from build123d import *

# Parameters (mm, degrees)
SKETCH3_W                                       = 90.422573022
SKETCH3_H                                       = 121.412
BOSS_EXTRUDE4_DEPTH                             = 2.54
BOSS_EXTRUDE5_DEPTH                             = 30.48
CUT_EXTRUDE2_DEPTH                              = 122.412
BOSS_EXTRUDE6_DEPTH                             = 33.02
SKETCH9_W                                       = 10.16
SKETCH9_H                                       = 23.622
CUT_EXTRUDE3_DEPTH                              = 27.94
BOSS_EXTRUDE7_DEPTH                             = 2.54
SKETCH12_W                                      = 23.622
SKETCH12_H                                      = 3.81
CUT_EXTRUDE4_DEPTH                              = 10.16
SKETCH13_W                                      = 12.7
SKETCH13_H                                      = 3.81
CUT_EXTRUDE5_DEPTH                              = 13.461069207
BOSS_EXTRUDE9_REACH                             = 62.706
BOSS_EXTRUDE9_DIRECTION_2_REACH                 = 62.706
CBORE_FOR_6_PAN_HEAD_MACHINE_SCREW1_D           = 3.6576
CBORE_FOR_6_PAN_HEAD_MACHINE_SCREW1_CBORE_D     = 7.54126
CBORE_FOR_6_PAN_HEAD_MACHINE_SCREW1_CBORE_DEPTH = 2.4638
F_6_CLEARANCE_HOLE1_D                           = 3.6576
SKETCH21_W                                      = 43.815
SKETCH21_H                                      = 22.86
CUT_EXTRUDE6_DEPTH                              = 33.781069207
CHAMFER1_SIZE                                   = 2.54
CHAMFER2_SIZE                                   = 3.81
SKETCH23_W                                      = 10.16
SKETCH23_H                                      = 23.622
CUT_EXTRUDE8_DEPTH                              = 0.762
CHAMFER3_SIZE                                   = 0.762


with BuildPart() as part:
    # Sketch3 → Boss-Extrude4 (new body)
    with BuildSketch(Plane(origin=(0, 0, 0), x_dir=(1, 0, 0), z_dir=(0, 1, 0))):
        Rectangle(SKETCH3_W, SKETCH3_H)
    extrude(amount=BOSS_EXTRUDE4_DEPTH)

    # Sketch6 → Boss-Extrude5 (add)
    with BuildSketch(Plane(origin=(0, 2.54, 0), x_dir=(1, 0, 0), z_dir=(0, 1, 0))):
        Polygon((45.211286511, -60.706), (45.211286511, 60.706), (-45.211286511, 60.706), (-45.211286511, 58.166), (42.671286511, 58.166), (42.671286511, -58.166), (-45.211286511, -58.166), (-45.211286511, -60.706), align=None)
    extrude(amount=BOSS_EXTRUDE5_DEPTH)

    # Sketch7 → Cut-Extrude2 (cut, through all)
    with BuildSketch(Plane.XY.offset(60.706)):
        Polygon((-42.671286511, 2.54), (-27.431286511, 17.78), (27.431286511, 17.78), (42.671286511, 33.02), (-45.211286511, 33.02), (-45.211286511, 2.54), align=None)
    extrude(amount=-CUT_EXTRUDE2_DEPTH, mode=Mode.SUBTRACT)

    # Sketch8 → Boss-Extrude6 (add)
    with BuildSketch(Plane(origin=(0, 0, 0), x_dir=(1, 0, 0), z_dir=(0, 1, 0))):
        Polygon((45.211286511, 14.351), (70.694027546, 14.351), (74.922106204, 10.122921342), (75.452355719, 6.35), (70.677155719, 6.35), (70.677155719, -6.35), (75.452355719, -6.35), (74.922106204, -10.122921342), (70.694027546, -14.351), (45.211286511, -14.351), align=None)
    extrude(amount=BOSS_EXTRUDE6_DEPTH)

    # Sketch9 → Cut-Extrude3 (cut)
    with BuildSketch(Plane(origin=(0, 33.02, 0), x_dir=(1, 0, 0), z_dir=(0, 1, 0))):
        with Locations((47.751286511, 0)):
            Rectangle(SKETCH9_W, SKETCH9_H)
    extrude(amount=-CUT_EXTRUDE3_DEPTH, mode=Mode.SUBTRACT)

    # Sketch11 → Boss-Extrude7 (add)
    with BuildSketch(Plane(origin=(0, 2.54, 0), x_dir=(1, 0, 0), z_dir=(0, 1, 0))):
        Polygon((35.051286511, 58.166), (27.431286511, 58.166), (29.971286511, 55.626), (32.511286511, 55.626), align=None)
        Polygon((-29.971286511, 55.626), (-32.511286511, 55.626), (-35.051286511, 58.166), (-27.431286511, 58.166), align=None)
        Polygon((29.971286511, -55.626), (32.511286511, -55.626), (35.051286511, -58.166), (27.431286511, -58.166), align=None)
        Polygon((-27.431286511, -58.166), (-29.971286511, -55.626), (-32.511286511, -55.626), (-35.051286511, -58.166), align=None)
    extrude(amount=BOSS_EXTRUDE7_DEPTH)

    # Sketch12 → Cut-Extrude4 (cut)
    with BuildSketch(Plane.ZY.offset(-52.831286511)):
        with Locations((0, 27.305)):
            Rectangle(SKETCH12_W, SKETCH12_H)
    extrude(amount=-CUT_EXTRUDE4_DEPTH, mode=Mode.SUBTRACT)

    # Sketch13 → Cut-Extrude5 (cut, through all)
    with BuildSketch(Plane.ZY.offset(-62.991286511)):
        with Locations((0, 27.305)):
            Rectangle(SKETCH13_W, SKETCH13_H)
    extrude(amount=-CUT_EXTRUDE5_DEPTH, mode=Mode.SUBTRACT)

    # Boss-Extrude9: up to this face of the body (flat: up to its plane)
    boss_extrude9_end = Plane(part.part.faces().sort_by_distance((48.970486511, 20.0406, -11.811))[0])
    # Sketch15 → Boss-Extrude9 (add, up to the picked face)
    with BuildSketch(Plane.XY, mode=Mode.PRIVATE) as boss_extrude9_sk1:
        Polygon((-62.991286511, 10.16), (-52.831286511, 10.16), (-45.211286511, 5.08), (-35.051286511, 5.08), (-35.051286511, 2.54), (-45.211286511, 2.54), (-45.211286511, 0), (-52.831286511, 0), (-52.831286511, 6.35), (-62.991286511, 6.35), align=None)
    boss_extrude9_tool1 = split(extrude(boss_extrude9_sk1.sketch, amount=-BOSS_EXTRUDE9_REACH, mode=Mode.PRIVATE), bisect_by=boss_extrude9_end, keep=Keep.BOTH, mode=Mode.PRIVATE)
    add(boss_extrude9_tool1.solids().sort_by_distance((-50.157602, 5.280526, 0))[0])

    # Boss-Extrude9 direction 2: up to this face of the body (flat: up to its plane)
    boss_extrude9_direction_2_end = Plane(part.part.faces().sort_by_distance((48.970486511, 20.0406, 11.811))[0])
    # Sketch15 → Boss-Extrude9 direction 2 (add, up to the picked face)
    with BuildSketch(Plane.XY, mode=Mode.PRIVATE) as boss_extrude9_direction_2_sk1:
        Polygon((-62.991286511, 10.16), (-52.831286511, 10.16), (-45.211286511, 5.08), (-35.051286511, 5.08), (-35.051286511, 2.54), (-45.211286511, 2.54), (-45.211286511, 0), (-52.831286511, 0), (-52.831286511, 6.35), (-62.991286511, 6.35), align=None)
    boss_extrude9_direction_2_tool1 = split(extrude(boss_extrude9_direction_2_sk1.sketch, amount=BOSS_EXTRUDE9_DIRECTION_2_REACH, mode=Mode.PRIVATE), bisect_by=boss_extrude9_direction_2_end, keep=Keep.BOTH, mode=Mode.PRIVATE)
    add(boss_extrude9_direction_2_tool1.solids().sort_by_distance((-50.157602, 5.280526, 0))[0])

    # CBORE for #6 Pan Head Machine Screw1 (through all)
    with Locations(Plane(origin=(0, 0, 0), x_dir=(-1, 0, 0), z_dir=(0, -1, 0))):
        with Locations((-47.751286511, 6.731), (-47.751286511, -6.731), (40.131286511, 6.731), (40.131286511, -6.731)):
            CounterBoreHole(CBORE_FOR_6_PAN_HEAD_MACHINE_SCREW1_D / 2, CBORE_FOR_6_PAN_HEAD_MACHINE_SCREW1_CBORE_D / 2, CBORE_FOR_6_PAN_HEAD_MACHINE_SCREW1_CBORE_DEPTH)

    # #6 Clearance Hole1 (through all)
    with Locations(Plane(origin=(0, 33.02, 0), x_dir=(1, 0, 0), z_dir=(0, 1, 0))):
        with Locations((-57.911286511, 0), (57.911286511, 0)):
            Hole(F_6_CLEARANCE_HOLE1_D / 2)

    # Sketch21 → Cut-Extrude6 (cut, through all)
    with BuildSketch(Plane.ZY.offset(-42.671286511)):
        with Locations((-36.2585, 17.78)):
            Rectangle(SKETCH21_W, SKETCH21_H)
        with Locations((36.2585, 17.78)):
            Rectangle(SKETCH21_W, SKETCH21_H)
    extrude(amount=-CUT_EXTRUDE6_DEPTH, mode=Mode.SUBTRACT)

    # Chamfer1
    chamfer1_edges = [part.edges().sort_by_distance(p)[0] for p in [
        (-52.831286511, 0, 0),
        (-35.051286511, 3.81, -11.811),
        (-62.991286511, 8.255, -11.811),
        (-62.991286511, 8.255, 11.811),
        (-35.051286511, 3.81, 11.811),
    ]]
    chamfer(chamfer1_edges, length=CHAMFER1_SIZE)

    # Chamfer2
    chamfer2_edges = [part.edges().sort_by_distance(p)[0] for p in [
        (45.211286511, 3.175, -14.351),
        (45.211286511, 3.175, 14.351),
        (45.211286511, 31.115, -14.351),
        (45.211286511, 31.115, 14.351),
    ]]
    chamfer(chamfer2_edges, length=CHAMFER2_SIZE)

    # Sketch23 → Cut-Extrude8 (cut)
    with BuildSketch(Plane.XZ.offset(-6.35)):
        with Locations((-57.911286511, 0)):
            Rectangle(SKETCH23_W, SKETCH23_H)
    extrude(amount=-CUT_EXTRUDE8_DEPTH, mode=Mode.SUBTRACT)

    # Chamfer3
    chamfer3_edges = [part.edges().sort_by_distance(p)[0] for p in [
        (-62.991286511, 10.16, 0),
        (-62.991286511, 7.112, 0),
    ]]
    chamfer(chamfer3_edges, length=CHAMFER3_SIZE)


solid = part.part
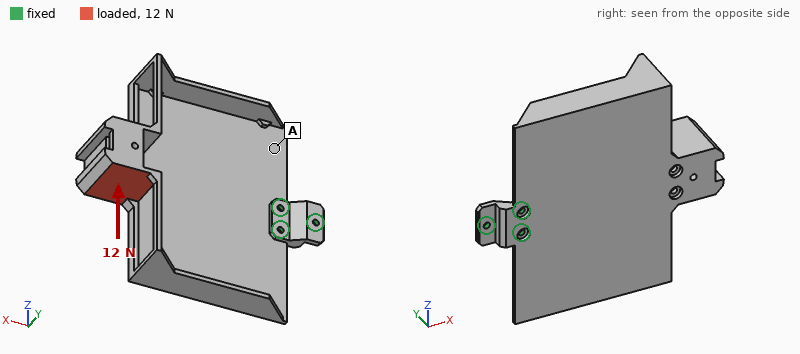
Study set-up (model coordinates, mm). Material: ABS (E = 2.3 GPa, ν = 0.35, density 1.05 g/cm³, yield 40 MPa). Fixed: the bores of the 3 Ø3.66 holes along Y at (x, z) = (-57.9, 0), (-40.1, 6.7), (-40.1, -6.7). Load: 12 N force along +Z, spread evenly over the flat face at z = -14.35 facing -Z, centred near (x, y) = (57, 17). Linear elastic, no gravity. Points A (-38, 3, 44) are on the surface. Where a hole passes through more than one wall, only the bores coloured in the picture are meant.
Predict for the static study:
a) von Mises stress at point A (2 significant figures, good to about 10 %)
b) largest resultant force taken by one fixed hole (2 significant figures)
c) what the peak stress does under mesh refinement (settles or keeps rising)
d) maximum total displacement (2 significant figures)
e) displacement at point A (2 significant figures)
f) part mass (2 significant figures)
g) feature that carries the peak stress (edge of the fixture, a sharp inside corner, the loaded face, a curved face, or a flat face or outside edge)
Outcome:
0.57 MPa
49 N
keeps rising
1.9 mm
0.40 mm
62 g
edge of the fixture
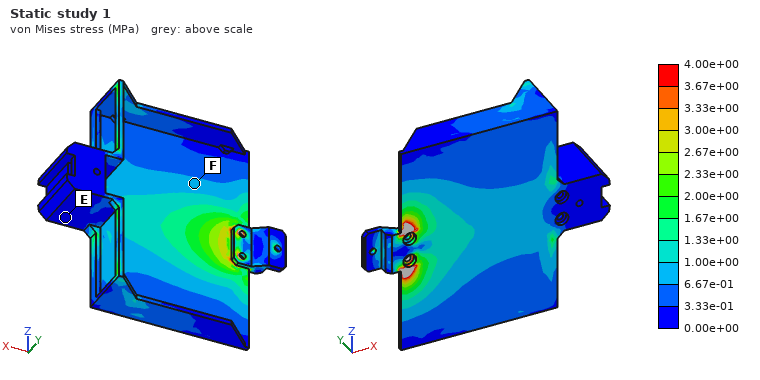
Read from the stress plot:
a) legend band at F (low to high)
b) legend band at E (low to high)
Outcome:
6.67e-01 to 1.00e+00 MPa
0.00e+00 to 3.33e-01 MPa
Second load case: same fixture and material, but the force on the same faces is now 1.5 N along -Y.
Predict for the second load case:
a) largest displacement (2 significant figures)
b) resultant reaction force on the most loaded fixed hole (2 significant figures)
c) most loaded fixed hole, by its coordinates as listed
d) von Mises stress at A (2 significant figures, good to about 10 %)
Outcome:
1.8 mm
7.4 N
(-57.9, 0)
0.70 MPa
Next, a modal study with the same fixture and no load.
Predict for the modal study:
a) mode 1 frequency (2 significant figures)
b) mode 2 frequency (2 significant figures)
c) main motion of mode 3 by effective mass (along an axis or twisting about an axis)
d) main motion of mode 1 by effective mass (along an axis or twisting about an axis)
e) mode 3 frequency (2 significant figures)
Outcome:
30 Hz
63 Hz
along Y
along Y
160 Hz
